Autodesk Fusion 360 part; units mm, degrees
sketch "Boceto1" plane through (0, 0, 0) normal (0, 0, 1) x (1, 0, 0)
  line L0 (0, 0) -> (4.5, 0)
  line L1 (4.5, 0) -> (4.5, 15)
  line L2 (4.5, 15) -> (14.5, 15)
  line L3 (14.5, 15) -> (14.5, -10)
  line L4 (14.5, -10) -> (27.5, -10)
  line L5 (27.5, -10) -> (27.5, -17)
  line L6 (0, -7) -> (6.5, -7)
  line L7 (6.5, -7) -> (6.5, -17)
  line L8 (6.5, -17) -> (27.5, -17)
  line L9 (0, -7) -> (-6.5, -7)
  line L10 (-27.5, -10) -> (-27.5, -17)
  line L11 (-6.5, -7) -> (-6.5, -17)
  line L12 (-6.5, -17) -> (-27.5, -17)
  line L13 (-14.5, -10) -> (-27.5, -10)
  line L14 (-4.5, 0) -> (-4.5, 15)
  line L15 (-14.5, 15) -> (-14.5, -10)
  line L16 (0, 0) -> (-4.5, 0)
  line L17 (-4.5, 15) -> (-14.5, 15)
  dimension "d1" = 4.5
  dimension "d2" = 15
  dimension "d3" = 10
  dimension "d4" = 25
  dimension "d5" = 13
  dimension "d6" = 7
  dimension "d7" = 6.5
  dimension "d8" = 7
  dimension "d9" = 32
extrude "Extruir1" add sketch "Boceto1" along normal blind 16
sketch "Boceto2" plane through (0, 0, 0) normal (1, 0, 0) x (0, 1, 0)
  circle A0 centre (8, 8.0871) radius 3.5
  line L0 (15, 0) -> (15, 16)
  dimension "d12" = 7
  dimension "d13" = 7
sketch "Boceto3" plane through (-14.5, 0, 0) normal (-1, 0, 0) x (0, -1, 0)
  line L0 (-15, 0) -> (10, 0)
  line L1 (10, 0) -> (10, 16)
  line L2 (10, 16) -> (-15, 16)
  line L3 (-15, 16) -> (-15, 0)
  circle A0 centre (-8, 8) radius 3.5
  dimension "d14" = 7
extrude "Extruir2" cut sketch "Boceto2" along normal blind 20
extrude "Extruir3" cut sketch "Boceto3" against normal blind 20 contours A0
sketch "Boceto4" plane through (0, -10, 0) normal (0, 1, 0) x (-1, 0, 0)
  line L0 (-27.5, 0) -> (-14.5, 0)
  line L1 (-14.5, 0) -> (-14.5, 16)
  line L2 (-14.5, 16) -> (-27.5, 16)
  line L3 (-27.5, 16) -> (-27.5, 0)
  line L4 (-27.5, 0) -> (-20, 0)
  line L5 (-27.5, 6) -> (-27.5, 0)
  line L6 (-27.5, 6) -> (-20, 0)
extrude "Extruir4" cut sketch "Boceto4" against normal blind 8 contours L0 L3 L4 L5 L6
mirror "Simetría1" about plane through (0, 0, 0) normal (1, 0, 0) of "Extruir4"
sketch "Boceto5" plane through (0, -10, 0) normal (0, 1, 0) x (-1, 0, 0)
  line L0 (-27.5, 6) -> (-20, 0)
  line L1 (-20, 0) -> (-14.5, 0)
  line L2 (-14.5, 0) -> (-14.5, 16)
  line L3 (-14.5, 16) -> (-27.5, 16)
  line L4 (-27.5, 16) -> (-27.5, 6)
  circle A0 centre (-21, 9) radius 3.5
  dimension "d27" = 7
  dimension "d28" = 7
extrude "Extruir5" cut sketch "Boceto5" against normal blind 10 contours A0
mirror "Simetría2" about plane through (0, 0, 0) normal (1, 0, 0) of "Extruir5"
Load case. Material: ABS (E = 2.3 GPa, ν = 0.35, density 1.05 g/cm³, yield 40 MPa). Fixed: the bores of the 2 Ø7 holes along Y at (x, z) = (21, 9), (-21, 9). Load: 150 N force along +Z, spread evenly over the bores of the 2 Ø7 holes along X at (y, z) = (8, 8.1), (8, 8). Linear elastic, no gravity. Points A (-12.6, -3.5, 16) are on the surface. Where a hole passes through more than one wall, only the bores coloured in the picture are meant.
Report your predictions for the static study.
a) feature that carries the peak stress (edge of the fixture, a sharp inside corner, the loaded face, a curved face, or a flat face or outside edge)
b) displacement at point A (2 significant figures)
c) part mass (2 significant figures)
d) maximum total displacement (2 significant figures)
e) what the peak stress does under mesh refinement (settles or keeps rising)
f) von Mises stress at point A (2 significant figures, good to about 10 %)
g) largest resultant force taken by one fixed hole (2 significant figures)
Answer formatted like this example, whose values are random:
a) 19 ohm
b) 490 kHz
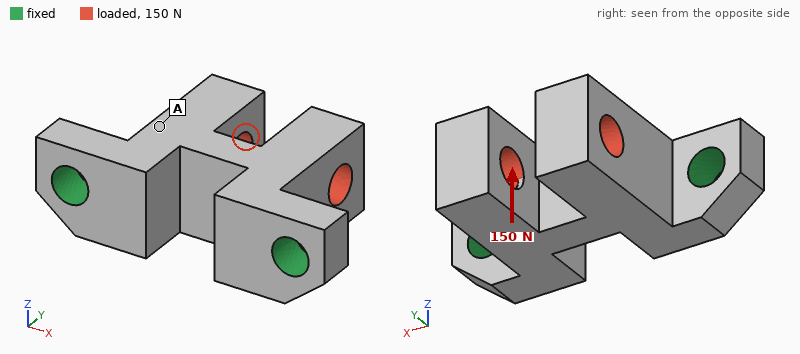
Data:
a) edge of the fixture
b) 0.12 mm
c) 12 g
d) 0.30 mm
e) keeps rising
f) 2.7 MPa
g) 75 N
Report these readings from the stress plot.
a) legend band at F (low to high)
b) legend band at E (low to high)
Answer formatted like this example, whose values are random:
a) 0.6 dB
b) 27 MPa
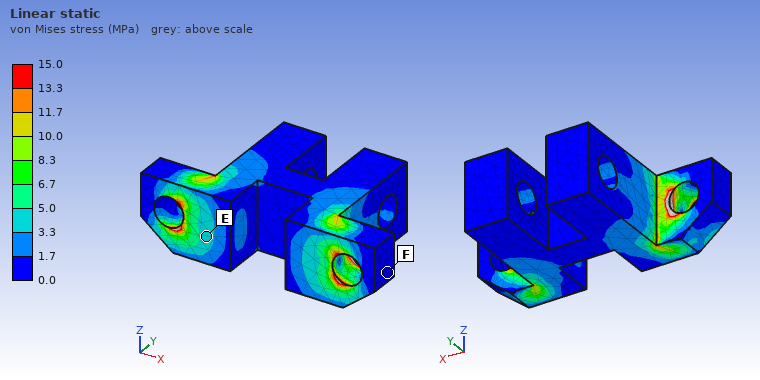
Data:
a) 0.0 to 1.7 MPa
b) 3.3 to 5.0 MPa
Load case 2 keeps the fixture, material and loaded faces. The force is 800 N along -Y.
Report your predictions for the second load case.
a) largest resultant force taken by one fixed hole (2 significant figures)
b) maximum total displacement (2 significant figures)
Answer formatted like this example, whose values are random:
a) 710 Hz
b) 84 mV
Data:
a) 450 N
b) 0.10 mm
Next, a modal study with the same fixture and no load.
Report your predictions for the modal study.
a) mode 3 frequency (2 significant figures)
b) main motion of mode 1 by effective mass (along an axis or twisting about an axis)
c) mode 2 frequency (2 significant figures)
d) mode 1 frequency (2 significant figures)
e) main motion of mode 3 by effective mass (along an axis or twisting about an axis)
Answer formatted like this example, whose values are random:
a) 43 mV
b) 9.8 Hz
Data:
a) 3800 Hz
b) along Z
c) 3300 Hz
d) 1800 Hz
e) along X
